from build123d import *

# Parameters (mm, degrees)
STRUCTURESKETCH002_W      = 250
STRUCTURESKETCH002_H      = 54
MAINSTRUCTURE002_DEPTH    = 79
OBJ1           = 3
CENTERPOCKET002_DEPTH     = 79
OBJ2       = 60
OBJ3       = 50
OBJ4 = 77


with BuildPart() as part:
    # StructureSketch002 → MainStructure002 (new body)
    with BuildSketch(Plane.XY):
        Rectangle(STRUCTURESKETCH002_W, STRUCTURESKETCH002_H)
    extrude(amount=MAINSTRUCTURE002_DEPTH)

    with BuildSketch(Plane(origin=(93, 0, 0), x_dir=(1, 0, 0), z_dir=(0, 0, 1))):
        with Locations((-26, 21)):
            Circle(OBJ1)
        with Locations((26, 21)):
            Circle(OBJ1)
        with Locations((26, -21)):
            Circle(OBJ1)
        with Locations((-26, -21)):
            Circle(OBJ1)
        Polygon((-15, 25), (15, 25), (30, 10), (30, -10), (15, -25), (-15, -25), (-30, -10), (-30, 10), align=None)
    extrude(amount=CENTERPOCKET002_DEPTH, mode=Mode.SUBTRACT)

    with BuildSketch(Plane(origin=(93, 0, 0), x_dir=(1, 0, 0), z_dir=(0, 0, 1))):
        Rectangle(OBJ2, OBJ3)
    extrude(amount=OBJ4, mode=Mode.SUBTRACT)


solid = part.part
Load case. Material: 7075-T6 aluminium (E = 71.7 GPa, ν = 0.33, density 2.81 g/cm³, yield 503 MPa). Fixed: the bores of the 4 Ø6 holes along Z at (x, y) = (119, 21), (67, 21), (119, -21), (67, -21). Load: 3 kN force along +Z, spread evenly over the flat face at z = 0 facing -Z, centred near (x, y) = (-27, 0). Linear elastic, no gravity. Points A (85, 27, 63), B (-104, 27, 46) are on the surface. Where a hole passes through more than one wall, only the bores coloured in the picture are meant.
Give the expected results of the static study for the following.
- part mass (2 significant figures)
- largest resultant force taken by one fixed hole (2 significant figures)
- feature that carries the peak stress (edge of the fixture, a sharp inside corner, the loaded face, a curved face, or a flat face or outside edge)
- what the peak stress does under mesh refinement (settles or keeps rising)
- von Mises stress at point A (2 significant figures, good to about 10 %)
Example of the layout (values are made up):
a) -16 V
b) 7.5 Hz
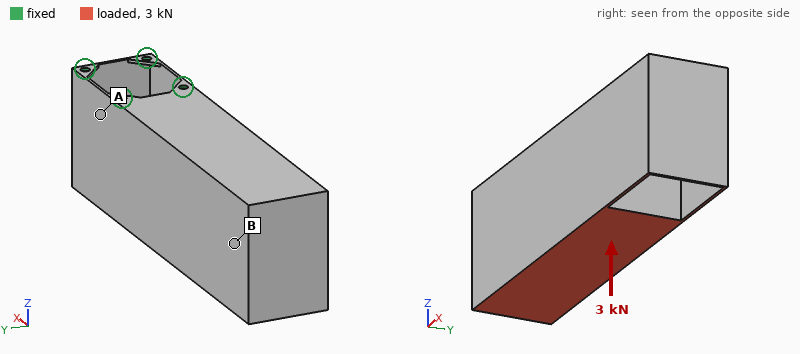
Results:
a) 2.3 kg
b) 4.1 kN
c) edge of the fixture
d) keeps rising
e) 40 MPa
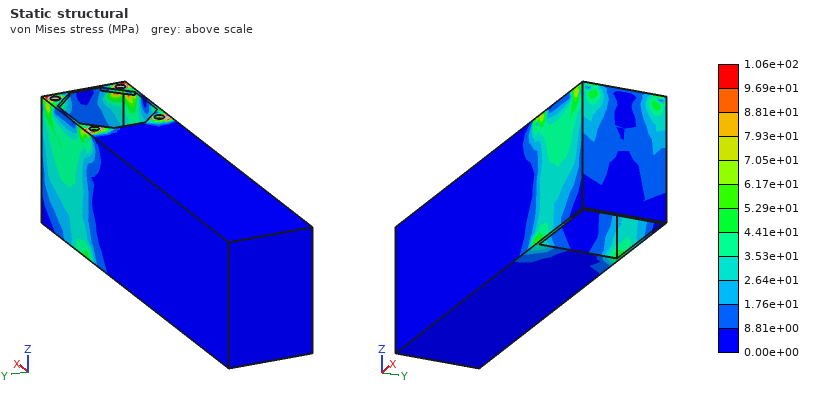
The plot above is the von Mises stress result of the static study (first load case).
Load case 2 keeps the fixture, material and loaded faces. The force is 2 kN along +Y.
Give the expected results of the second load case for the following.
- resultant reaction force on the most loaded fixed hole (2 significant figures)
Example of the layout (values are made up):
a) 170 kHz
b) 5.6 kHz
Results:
a) 4.5 kN
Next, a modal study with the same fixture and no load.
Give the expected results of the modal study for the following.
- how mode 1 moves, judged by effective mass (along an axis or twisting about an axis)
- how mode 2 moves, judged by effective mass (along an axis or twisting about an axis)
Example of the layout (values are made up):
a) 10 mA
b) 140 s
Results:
a) along Z
b) along Y
